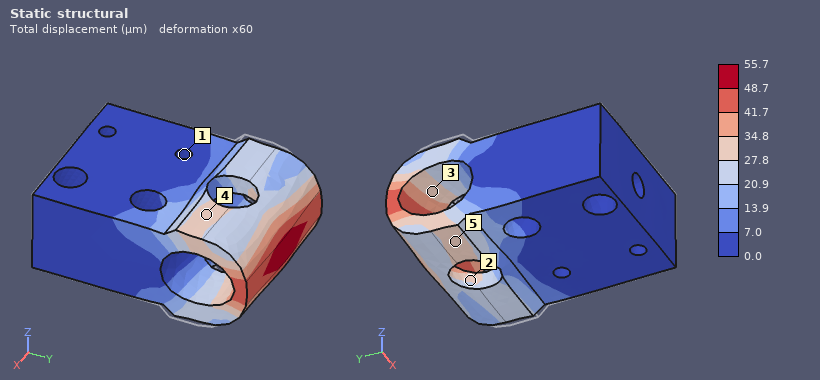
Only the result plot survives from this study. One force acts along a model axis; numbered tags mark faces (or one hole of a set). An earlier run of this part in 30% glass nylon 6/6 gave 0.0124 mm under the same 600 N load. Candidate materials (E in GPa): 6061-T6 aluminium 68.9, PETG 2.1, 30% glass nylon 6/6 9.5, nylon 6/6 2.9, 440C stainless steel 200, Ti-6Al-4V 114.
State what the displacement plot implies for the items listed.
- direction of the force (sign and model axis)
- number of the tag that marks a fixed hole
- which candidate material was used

+Y
1
PETG
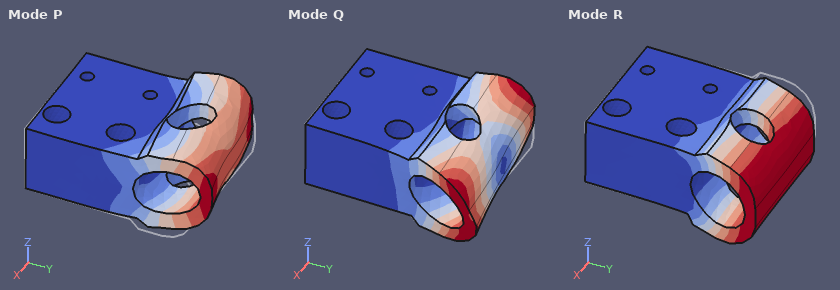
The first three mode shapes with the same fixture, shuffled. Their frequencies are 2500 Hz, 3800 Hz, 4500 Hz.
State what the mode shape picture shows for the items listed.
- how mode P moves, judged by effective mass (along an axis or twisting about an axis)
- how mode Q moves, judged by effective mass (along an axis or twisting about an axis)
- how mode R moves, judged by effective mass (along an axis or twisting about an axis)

along X
twisting about Y
along Z
